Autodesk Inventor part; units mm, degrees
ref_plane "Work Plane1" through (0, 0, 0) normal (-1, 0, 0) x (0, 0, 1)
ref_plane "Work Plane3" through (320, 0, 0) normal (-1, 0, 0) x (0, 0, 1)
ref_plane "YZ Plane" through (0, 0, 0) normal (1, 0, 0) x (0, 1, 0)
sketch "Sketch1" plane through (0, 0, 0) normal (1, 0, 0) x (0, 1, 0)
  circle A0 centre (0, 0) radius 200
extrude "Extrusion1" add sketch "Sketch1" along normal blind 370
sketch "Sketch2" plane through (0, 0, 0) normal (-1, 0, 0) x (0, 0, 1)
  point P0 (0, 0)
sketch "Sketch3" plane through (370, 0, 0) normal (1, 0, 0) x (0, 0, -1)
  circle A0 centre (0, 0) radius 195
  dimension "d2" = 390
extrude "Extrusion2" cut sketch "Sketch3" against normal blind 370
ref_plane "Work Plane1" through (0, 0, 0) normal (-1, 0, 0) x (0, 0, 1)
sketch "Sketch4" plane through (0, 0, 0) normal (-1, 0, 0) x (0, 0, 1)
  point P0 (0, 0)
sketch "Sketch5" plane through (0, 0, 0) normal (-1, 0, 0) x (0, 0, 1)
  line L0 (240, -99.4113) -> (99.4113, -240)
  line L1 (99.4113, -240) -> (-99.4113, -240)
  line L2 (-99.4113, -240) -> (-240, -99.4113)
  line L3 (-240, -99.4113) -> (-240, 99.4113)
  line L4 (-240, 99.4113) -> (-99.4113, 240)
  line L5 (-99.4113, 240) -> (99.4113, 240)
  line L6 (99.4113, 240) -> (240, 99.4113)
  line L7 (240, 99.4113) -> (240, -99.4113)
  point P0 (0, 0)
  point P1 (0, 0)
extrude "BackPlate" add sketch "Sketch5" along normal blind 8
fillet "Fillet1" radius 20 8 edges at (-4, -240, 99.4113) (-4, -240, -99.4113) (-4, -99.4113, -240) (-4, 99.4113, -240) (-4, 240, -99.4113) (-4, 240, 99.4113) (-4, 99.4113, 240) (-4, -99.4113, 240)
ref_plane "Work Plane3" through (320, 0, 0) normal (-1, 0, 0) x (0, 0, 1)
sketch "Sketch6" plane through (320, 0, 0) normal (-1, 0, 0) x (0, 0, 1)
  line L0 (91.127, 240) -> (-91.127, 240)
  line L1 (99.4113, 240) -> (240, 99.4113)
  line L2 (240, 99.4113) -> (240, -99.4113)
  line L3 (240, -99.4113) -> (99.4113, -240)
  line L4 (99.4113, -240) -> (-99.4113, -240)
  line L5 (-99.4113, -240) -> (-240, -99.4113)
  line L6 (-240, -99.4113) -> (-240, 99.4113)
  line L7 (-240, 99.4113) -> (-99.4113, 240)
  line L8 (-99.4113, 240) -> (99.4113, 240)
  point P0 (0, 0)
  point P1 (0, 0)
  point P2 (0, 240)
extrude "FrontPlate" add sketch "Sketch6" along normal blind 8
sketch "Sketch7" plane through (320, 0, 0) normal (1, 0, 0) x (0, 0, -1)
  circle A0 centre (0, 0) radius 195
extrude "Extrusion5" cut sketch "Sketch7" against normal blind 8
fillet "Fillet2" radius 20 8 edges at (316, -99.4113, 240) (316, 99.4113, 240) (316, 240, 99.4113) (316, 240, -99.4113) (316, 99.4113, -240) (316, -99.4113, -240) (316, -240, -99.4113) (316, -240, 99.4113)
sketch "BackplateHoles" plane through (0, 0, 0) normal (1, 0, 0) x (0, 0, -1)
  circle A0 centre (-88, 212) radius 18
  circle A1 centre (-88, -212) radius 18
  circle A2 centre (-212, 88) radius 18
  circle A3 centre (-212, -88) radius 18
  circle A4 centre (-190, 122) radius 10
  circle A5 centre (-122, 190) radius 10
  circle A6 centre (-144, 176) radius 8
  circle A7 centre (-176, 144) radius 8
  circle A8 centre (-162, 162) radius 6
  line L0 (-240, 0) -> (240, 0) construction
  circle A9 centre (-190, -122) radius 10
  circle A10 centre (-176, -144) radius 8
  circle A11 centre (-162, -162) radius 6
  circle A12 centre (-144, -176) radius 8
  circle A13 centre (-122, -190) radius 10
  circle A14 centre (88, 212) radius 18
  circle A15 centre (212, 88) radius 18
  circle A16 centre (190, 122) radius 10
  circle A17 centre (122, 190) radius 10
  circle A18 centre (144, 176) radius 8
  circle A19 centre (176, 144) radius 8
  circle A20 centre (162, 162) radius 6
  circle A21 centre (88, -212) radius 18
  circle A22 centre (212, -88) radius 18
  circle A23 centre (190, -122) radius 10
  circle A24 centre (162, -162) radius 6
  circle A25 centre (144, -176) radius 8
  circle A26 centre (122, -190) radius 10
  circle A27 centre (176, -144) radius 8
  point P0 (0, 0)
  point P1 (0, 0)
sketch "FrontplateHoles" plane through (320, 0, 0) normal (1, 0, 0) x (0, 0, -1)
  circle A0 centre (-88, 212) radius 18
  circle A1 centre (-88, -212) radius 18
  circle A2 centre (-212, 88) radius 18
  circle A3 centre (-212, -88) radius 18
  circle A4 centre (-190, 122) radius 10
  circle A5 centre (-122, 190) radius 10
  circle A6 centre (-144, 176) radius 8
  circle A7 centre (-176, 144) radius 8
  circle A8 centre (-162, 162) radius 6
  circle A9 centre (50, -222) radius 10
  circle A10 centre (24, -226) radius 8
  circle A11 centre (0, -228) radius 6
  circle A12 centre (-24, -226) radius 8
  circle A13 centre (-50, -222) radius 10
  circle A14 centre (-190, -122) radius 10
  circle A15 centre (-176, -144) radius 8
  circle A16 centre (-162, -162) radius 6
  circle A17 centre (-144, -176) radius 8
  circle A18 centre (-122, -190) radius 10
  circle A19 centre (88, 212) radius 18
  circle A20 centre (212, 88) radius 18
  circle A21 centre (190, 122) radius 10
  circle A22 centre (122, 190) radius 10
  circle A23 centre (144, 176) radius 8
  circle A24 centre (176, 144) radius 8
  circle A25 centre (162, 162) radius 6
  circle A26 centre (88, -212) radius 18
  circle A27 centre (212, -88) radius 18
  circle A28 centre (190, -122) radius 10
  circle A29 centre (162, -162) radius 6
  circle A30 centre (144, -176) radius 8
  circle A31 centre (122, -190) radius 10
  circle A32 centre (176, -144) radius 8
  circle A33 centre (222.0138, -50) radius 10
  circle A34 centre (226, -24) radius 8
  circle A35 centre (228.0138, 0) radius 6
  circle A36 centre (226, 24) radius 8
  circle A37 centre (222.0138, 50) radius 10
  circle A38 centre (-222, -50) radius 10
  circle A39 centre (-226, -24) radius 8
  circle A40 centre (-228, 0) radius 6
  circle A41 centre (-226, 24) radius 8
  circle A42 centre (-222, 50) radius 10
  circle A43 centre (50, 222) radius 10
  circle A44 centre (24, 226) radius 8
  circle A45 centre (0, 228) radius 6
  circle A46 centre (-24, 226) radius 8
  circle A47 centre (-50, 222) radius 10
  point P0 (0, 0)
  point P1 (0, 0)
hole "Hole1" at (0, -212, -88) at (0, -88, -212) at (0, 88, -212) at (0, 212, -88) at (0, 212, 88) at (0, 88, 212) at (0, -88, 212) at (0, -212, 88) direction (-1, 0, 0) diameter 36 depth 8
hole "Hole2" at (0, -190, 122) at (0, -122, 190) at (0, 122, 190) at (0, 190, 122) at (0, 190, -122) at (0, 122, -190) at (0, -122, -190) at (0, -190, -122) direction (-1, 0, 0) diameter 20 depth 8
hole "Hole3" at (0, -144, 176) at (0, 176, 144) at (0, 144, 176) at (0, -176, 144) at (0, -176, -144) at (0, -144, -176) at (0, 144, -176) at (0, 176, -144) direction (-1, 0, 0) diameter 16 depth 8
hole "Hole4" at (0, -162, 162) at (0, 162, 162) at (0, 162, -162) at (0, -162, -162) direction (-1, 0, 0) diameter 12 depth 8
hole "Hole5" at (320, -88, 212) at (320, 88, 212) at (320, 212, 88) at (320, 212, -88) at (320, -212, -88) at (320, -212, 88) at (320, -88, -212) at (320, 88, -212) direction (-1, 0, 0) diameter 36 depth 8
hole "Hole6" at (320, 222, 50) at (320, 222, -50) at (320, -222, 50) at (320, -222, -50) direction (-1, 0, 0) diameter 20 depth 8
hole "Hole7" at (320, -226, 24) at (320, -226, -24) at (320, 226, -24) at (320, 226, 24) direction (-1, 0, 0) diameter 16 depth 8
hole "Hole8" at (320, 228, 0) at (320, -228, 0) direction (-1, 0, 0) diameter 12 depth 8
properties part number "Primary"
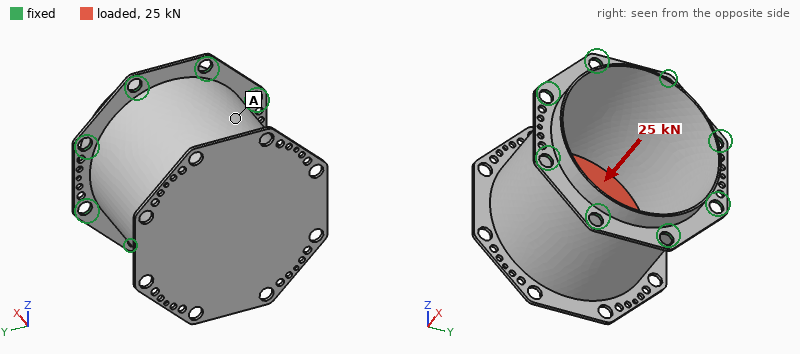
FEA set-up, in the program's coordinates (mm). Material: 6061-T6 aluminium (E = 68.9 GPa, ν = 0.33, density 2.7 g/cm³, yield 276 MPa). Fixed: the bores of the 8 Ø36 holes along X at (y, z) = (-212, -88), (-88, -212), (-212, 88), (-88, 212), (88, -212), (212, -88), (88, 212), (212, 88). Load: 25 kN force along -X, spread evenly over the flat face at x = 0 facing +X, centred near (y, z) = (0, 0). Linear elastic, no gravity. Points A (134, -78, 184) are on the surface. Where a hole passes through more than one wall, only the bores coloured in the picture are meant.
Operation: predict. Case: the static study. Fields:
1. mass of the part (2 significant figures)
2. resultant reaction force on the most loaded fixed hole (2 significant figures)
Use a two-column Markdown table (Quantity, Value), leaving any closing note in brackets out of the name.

| Quantity | Value |
|---|---|
| mass of the part | 11 kg |
| resultant reaction force on the most loaded fixed hole | 3.2 kN |
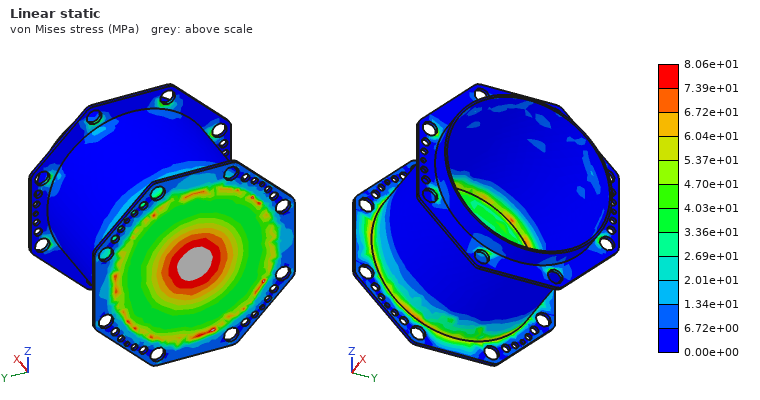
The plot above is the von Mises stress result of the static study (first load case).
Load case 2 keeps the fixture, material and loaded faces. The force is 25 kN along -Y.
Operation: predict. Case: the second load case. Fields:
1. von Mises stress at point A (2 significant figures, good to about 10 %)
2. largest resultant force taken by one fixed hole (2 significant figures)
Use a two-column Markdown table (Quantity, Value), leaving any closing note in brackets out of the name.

| Quantity | Value |
|---|---|
| von Mises stress at point A | 13 MPa |
| largest resultant force taken by one fixed hole | 9.2 kN |
